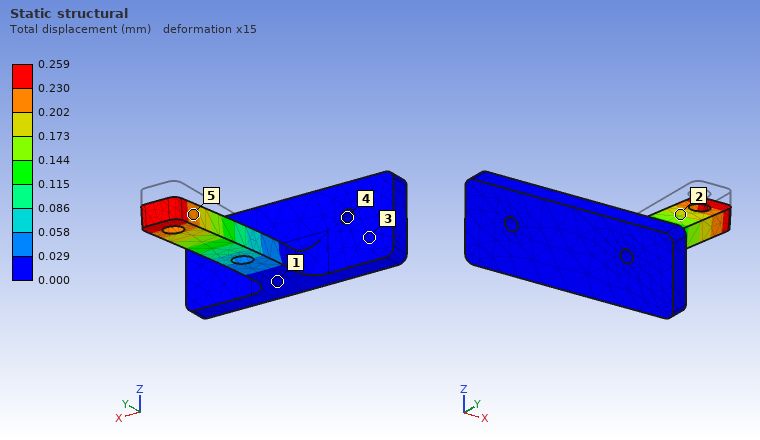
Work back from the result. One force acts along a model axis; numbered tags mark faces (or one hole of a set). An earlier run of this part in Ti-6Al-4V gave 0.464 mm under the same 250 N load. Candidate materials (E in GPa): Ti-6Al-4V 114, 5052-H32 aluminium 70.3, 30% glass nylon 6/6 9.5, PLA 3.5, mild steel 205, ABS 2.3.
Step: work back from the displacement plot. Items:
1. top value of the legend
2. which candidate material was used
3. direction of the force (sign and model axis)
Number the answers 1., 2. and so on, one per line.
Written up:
1. 0.259 mm
2. mild steel
3. -Z
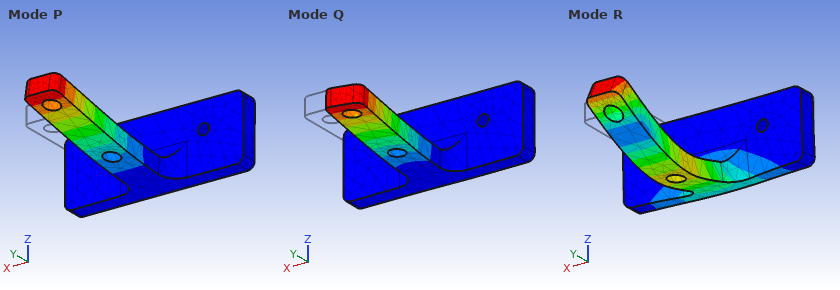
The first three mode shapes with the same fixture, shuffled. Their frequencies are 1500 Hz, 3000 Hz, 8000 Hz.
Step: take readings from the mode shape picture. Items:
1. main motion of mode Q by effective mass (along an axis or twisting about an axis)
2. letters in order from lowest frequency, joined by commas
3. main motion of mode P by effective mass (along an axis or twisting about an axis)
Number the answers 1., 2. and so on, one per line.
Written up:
1. along X
2. P, Q, R
3. along Z
